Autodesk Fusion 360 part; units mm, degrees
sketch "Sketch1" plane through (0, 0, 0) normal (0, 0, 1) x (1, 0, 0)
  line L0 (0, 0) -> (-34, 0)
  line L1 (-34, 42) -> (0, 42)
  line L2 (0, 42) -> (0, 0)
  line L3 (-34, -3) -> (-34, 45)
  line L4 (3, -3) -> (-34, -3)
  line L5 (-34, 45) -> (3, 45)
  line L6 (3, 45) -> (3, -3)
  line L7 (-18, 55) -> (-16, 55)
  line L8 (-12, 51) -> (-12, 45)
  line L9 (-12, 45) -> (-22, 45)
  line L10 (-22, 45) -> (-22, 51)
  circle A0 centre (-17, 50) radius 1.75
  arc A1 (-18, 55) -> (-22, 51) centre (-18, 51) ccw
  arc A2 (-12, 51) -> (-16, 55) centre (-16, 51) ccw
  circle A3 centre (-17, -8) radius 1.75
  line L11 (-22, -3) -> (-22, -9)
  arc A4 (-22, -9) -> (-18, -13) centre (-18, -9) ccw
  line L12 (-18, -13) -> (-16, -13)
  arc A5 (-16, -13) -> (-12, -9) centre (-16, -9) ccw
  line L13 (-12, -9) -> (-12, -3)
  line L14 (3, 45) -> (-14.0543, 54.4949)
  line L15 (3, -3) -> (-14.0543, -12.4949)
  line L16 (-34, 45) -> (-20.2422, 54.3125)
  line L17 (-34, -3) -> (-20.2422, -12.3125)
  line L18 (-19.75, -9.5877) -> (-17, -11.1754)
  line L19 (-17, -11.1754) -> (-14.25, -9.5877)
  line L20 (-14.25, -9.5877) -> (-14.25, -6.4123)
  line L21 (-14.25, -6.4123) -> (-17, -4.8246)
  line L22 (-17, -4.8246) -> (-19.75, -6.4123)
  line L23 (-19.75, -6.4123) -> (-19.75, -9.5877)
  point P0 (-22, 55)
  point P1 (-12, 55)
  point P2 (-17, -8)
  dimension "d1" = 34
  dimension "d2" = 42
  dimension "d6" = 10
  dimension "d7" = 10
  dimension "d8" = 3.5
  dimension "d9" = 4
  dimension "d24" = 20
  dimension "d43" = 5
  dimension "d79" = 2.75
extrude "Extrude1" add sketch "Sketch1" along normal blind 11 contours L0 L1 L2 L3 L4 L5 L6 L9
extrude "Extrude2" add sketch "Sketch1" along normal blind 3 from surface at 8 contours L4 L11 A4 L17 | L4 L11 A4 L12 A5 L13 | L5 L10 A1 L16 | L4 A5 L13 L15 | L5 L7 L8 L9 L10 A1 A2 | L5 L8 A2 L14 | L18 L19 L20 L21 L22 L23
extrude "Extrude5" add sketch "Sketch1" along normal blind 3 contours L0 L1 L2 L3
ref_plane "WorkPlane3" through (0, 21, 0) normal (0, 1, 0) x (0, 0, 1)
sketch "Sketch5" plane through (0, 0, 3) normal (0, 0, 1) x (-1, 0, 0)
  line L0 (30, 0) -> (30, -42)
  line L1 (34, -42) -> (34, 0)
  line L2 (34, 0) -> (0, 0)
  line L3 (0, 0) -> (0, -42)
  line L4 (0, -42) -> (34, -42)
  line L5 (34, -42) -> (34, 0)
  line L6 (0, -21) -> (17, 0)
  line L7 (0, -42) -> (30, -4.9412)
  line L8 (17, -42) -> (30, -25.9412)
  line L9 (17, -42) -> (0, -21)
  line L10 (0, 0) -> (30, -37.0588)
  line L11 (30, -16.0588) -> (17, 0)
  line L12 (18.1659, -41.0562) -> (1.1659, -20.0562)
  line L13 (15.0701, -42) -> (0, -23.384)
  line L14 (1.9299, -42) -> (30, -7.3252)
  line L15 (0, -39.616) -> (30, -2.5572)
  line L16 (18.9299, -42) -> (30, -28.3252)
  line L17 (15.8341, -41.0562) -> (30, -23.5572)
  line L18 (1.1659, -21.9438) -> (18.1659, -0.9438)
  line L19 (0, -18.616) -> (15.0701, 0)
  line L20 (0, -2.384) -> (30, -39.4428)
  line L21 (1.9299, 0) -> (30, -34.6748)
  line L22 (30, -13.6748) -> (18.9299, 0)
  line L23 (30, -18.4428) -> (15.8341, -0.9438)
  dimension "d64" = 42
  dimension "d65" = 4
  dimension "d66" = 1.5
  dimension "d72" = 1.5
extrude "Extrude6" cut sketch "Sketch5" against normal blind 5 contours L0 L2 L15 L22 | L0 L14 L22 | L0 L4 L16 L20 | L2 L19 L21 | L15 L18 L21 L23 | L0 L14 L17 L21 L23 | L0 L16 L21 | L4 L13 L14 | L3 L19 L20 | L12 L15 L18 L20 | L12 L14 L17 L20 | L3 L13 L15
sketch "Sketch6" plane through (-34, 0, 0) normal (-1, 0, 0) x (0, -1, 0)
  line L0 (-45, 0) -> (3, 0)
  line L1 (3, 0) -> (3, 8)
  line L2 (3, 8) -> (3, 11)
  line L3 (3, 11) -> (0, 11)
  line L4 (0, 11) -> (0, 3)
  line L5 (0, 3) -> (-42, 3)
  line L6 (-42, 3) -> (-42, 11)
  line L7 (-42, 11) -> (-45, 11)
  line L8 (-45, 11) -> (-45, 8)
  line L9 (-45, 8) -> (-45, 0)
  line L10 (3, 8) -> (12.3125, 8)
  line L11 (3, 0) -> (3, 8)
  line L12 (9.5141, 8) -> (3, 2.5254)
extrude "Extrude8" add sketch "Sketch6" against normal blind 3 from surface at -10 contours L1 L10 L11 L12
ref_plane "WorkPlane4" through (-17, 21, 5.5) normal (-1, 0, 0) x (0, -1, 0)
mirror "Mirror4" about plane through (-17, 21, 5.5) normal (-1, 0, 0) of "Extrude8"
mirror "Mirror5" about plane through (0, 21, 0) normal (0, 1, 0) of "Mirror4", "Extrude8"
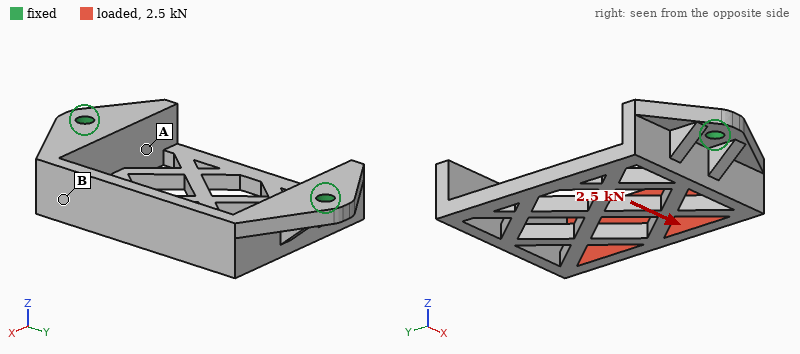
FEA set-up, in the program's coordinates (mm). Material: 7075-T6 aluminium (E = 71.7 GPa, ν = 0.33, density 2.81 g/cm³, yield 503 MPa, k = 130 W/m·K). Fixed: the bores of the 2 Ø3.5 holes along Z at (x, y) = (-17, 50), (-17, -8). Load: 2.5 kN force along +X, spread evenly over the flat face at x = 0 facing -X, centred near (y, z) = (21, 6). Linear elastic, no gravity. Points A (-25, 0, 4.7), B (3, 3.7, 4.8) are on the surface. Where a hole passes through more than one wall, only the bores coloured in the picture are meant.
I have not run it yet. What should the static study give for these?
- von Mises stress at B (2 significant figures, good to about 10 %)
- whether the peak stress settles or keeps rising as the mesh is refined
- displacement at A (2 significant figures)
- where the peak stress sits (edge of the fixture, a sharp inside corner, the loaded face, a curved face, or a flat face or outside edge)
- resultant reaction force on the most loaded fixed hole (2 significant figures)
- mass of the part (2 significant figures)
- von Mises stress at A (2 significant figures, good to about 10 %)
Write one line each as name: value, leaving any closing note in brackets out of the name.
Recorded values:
von Mises stress at B: 89 MPa
whether the peak stress settles or keeps rising as the mesh is refined: keeps rising
displacement at A: 0.037 mm
where the peak stress sits: edge of the fixture
resultant reaction force on the most loaded fixed hole: 1.4 kN
mass of the part: 20 g
von Mises stress at A: 33 MPa
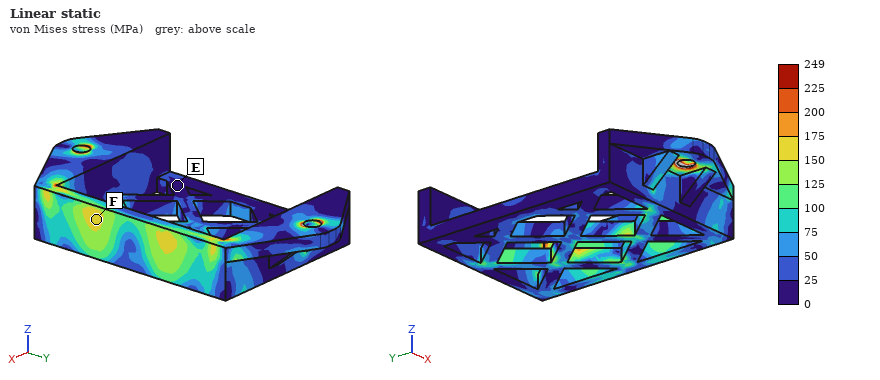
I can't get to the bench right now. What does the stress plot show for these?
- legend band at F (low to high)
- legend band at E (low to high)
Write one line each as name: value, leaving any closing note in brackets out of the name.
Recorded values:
legend band at F: 150 to 175 MPa
legend band at E: 0 to 25 MPa
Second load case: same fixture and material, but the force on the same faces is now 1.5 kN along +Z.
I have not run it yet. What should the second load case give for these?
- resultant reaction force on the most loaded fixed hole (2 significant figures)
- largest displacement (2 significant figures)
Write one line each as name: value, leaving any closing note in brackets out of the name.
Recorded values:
resultant reaction force on the most loaded fixed hole: 840 N
largest displacement: 0.39 mm
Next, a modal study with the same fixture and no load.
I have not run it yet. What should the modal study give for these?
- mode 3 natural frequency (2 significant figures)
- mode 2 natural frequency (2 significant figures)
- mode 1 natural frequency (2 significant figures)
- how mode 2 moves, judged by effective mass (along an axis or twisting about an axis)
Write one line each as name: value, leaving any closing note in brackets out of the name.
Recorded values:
mode 3 natural frequency: 6600 Hz
mode 2 natural frequency: 5800 Hz
mode 1 natural frequency: 3600 Hz
how mode 2 moves, judged by effective mass: along Z
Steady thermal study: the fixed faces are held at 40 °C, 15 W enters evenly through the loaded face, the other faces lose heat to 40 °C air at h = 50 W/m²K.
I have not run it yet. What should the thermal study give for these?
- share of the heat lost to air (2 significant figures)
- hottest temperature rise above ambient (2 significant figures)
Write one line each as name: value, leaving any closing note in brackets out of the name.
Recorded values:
share of the heat lost to air: 21 %
hottest temperature rise above ambient: 31 K
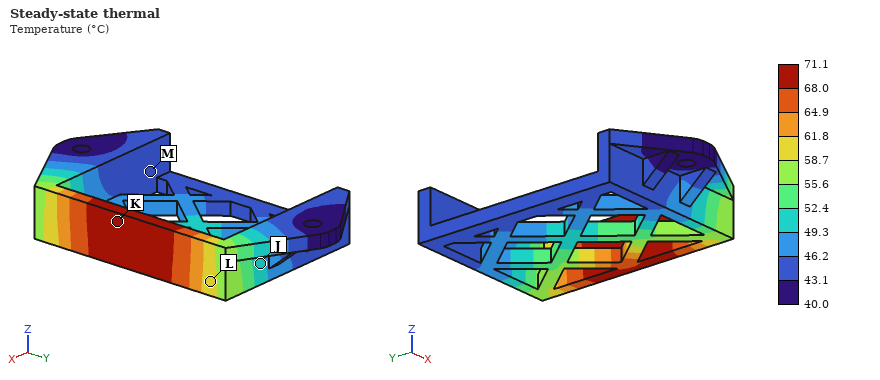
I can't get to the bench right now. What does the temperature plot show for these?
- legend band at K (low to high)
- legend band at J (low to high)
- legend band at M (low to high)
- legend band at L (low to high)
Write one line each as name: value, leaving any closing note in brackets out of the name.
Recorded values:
legend band at K: 68.0 to 71.1 °C
legend band at J: 49.3 to 52.4 °C
legend band at M: 43.1 to 46.2 °C
legend band at L: 58.7 to 61.8 °C
